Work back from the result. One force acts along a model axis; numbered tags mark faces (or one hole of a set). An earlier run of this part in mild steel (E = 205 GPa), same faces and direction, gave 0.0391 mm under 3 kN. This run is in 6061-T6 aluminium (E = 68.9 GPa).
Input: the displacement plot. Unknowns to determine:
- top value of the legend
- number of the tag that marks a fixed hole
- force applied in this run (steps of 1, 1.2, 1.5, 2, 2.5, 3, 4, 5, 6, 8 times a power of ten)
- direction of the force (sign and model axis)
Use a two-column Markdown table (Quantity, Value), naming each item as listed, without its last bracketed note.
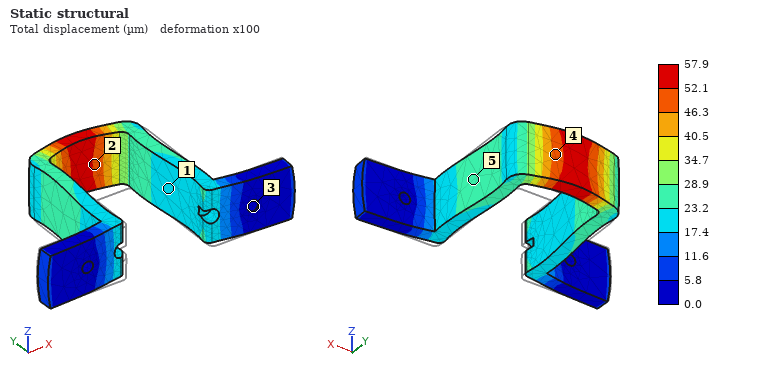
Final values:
| Quantity | Value |
|---|---|
| top value of the legend | 57.9 µm |
| number of the tag that marks a fixed hole | 3 |
| force applied in this run | 1.5 kN |
| direction of the force | +Y |
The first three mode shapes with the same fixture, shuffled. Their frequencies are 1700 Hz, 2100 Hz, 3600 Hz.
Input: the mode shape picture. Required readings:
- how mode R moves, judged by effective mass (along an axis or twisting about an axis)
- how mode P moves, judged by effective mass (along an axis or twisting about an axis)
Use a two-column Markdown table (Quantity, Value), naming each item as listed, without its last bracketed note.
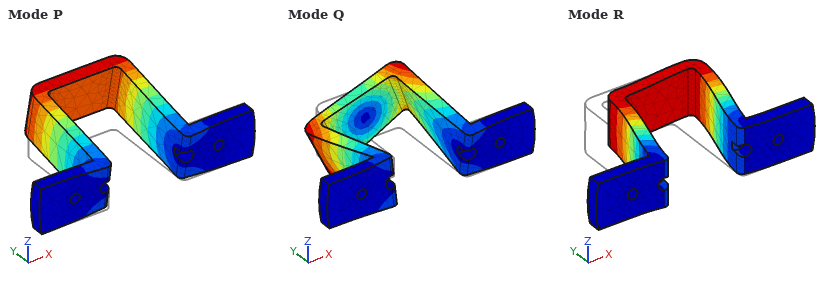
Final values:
| Quantity | Value |
|---|---|
| how mode R moves, judged by effective mass | along X |
| how mode P moves, judged by effective mass | along Z |
